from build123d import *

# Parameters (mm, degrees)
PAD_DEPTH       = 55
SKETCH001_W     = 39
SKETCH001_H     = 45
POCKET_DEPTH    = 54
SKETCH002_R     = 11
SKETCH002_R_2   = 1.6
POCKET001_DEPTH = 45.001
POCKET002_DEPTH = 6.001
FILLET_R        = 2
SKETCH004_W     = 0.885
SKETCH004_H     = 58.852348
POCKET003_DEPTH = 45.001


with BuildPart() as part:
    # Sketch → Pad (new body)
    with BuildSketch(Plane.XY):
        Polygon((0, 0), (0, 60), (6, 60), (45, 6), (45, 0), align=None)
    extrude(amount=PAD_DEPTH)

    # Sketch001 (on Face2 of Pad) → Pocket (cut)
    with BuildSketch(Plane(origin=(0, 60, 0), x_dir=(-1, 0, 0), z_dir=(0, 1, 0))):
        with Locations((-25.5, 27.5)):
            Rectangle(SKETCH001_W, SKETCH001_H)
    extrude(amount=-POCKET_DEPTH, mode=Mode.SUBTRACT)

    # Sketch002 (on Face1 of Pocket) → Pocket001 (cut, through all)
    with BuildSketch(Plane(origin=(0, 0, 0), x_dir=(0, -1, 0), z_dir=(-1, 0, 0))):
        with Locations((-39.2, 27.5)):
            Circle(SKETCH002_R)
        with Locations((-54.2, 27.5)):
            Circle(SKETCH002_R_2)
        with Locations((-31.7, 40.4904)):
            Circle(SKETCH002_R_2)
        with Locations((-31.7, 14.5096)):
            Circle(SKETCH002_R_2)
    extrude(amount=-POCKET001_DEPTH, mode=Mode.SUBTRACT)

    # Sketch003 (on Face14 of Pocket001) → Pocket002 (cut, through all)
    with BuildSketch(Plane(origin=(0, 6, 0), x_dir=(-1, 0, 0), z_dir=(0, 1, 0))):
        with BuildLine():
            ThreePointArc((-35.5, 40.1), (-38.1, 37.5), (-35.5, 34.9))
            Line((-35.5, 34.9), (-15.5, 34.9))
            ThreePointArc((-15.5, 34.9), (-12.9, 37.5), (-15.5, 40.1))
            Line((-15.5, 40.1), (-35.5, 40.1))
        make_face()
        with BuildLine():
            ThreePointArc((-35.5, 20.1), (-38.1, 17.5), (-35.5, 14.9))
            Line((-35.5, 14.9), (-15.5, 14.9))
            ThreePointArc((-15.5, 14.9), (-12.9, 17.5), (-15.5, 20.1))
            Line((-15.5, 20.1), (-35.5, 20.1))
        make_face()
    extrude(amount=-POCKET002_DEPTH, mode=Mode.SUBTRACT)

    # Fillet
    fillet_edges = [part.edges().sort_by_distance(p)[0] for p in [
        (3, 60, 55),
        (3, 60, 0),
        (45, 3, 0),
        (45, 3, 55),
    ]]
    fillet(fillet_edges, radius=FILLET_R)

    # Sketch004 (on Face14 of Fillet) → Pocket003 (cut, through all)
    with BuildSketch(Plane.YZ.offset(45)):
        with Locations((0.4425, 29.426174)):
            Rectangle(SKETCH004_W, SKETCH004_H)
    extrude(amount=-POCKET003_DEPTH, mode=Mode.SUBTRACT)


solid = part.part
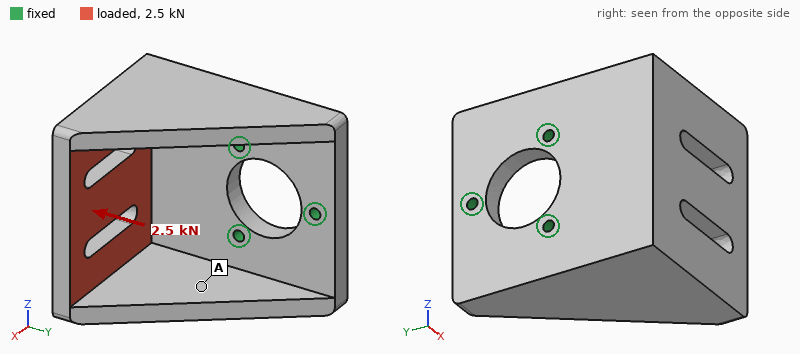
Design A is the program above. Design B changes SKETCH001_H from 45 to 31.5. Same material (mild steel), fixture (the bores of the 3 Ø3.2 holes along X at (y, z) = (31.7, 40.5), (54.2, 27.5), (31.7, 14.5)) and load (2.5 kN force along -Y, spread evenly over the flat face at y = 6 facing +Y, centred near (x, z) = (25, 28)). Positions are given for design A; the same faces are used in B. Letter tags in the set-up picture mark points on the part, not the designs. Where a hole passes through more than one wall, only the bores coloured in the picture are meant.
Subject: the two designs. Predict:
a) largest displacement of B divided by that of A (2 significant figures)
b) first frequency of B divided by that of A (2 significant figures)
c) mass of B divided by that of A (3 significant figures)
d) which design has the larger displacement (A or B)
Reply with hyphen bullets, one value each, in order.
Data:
- 0.48
- 1.2
- 1.38
- A
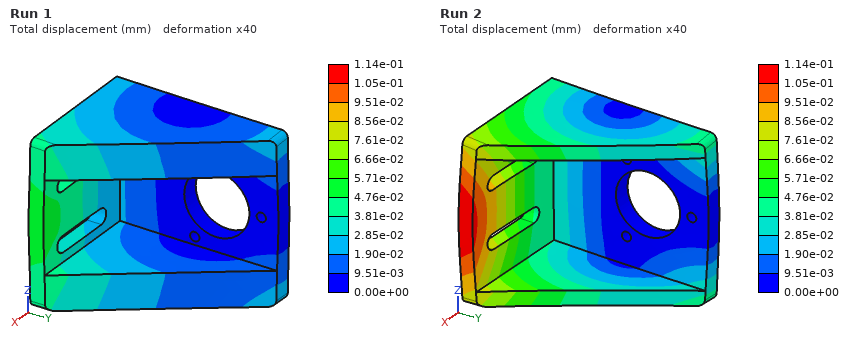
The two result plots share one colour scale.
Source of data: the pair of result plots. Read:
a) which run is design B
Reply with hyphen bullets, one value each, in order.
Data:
- Run 1
